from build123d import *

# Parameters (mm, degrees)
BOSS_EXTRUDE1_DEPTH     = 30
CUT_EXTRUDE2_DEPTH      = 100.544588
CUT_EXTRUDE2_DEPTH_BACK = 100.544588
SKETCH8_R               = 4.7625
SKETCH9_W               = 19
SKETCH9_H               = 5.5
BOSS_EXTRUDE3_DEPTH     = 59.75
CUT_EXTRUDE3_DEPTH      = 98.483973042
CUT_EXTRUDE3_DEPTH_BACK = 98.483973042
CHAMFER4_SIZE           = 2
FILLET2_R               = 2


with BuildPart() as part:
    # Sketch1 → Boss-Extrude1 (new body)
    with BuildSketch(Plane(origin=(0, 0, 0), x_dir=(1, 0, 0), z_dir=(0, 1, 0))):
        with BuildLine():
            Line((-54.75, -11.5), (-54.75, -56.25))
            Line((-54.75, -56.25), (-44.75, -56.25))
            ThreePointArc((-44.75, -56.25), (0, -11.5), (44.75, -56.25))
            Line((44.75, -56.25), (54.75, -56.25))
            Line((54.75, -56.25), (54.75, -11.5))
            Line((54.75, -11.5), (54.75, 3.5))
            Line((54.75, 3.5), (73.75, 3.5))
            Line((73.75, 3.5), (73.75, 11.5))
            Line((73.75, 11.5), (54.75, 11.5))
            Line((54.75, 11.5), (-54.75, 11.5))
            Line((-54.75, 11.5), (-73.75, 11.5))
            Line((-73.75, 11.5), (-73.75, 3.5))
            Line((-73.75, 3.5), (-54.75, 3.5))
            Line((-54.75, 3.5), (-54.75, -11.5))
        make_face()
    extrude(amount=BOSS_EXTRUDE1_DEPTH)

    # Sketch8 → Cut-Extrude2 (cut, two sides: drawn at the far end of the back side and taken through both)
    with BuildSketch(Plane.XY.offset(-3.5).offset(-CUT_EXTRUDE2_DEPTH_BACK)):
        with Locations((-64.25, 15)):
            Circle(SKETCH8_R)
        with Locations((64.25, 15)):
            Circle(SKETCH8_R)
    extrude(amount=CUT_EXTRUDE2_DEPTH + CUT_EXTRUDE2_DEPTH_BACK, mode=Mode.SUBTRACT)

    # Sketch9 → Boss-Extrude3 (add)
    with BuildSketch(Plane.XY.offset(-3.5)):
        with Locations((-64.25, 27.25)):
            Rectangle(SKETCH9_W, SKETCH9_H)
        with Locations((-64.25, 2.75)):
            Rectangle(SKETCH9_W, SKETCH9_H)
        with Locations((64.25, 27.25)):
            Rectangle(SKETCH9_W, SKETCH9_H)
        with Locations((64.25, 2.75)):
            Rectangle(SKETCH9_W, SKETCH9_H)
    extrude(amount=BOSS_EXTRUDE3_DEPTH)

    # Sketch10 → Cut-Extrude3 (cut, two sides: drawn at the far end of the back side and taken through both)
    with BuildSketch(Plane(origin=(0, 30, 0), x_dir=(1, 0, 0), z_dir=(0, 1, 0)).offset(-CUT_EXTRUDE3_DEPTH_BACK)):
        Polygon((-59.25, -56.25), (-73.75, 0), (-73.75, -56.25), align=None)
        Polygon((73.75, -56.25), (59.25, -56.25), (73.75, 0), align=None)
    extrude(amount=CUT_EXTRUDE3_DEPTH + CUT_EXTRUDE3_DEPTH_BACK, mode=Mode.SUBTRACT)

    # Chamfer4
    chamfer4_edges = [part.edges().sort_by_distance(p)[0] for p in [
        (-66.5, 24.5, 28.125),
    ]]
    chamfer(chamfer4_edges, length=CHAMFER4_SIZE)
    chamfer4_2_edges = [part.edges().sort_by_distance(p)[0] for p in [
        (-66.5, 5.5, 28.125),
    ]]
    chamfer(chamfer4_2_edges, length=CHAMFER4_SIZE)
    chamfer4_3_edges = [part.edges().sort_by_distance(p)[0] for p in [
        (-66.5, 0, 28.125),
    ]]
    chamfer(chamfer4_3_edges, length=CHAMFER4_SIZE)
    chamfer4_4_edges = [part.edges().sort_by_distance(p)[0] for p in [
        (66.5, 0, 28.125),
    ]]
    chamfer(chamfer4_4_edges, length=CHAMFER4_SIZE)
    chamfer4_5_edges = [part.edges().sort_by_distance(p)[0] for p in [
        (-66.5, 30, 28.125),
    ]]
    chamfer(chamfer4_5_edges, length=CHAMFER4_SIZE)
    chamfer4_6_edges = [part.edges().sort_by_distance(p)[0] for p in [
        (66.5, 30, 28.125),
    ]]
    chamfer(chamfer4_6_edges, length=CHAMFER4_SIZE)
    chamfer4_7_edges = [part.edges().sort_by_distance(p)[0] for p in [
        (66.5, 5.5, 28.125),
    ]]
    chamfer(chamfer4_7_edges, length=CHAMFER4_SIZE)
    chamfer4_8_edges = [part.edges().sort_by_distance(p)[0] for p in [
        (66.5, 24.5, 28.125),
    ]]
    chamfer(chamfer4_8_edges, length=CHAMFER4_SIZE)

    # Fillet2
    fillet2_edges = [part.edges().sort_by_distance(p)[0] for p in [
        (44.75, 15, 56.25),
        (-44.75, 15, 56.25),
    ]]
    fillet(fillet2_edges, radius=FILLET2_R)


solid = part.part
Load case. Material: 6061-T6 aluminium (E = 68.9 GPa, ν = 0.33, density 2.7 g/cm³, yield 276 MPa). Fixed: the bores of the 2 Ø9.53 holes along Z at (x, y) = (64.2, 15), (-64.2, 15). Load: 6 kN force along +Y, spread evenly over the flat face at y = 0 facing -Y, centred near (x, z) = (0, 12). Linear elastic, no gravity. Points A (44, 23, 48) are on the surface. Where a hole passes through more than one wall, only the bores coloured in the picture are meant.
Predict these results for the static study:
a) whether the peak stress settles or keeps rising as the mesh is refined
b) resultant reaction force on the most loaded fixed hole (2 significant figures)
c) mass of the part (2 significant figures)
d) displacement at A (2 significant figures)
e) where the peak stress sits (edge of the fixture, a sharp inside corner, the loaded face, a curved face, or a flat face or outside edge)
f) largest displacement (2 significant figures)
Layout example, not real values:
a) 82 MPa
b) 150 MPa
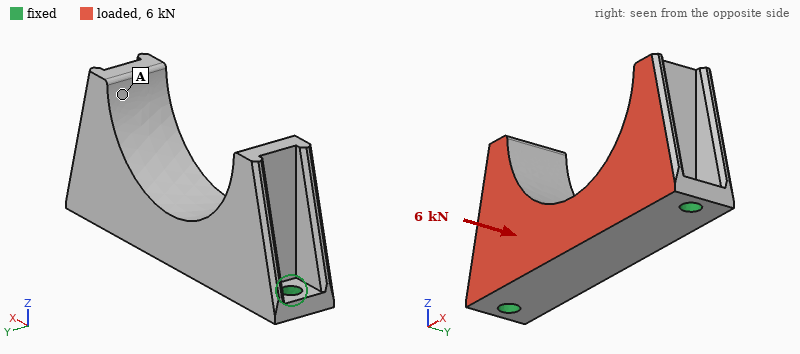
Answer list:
a) keeps rising
b) 3.0 kN
c) 410 g
d) 0.13 mm
e) edge of the fixture
f) 0.14 mm
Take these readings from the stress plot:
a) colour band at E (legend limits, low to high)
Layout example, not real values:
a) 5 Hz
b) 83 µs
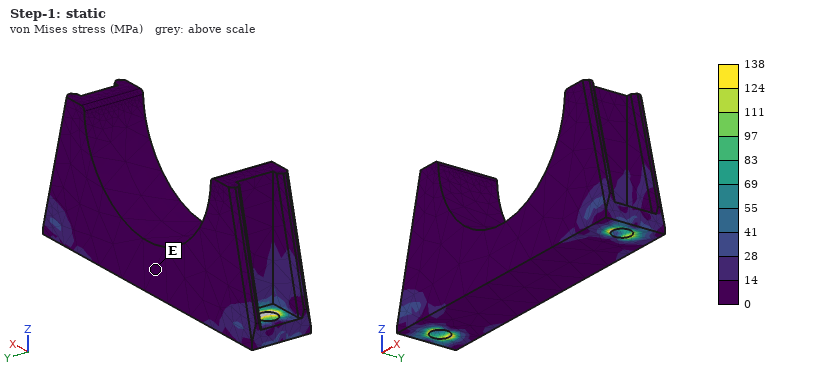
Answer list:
a) 0 to 14 MPa
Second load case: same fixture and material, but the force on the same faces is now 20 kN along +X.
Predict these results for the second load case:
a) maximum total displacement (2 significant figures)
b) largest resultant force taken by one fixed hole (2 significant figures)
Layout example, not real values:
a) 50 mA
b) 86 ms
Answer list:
a) 69 µm
b) 11 kN
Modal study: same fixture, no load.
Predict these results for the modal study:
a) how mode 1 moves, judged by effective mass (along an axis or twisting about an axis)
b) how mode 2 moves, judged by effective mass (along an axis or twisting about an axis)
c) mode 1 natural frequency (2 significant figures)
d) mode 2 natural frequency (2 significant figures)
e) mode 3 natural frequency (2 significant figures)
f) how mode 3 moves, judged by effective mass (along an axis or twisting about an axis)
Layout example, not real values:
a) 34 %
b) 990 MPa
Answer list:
a) along Y
b) along Z
c) 2100 Hz
d) 3600 Hz
e) 3800 Hz
f) twisting about Z
